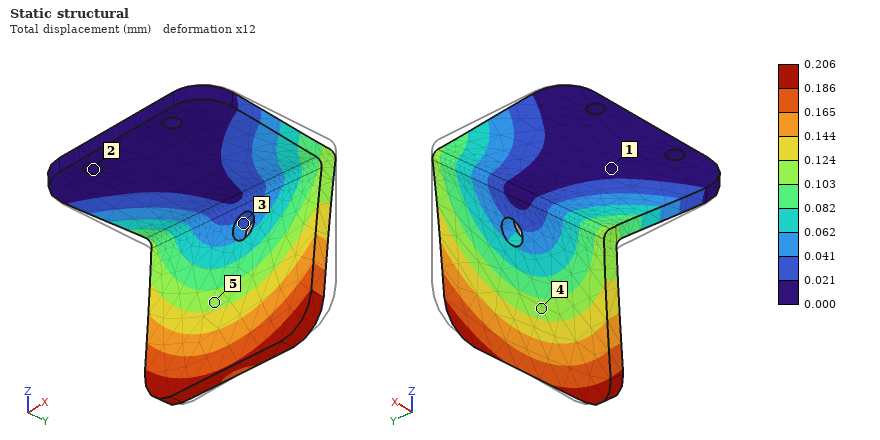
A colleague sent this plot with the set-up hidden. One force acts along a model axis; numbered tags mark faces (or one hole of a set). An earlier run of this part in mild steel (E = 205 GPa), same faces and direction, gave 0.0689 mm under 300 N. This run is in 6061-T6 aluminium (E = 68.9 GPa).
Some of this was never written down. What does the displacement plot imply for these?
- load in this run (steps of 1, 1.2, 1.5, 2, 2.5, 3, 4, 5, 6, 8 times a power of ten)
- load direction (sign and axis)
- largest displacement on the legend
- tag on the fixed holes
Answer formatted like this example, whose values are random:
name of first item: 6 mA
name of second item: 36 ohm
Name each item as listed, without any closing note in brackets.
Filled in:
load in this run: 300 N
load direction: -X
largest displacement on the legend: 0.206 mm
tag on the fixed holes: 2
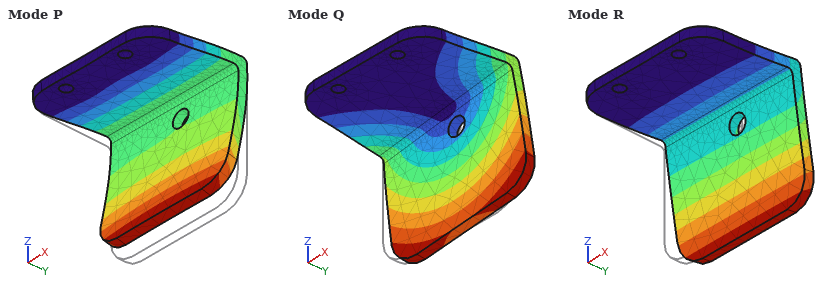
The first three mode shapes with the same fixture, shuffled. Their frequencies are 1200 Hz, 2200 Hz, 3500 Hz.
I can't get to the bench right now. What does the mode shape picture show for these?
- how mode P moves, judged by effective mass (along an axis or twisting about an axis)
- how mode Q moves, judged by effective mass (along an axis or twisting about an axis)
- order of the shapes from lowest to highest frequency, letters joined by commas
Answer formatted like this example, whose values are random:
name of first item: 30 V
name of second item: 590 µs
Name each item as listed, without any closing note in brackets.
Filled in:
how mode P moves, judged by effective mass: along Z
how mode Q moves, judged by effective mass: along X
order of the shapes from lowest to highest frequency, letters joined by commas: R, Q, P
